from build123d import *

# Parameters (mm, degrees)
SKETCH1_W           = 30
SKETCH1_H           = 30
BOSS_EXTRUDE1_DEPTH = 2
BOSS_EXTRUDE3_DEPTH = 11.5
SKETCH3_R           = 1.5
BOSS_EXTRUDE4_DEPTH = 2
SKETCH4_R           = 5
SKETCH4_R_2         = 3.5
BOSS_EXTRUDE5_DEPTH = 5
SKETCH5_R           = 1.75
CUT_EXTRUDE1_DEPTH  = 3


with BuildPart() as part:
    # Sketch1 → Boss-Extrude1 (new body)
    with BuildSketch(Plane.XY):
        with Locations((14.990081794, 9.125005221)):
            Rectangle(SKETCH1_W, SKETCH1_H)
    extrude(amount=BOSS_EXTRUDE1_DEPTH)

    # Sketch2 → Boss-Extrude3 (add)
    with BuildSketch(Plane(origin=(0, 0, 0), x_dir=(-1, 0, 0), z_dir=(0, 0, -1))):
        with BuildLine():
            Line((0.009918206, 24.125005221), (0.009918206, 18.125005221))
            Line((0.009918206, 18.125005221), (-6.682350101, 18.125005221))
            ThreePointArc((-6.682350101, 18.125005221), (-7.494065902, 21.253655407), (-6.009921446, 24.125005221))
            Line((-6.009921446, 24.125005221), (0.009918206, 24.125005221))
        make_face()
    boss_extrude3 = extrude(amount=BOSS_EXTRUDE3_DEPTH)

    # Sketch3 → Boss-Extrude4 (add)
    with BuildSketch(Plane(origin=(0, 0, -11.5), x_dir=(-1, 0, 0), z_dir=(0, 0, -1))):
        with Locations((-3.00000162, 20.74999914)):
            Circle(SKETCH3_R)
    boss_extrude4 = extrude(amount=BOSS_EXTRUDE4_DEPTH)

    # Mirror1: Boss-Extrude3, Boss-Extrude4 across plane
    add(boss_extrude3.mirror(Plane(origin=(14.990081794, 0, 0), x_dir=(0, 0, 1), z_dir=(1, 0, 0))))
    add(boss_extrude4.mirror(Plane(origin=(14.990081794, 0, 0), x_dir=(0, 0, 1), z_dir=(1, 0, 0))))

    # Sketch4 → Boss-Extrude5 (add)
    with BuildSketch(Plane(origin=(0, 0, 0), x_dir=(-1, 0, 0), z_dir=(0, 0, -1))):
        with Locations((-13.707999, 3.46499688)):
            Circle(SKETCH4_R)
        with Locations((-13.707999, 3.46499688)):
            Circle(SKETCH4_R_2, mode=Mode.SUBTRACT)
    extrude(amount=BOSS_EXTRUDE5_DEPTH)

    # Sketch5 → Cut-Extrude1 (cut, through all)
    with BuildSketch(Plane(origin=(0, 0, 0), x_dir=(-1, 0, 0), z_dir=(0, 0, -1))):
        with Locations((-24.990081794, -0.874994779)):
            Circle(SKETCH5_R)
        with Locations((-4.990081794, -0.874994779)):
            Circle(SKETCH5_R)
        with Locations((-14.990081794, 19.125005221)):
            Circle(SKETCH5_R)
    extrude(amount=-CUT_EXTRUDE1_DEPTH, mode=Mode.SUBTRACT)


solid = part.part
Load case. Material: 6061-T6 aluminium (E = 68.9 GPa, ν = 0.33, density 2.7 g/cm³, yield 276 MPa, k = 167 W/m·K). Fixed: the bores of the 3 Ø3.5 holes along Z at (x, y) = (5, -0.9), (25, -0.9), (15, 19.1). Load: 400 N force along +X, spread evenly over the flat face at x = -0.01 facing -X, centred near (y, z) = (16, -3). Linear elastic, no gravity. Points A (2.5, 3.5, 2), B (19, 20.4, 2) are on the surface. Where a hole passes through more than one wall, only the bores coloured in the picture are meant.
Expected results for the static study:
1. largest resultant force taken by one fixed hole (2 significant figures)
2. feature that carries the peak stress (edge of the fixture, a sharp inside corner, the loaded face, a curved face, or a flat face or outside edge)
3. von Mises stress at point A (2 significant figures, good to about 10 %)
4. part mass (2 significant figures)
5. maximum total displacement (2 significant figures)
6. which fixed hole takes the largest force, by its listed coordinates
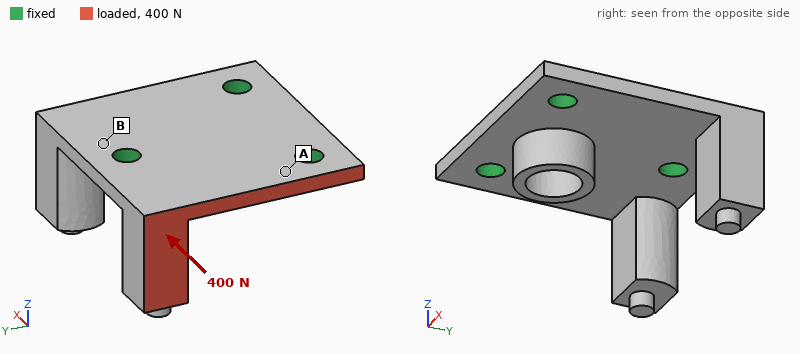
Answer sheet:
290 N
a flat face or outside edge
59 MPa
8.0 g
0.23 mm
(15, 19.1)
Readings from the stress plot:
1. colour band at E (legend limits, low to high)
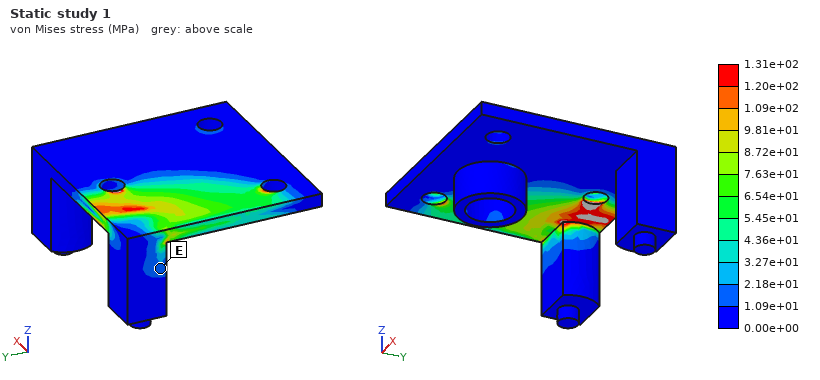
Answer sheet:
1.09e+01 to 2.18e+01 MPa
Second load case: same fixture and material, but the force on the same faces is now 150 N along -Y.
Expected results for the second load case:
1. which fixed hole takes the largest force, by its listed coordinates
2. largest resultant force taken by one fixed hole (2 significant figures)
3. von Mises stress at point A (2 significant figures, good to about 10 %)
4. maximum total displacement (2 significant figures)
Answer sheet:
(5, -0.9)
120 N
10 MPa
60 µm
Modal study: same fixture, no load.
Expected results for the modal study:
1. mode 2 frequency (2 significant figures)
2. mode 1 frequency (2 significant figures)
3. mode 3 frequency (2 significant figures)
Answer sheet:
3900 Hz
3800 Hz
6900 Hz
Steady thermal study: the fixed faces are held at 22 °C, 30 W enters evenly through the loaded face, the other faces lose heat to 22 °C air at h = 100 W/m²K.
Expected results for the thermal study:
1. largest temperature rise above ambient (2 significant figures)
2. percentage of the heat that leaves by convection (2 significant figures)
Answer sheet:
57 K
10.0 %
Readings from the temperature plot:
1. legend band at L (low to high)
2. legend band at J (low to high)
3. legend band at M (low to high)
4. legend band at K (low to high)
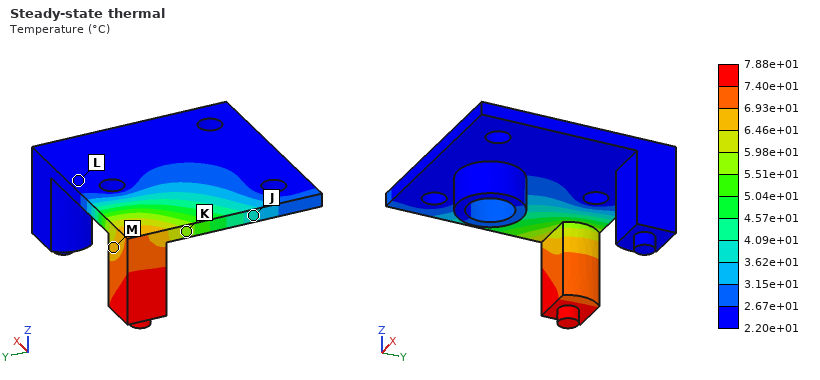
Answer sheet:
2.20e+01 to 2.67e+01 °C
3.62e+01 to 4.09e+01 °C
6.46e+01 to 6.93e+01 °C
5.51e+01 to 5.98e+01 °C
